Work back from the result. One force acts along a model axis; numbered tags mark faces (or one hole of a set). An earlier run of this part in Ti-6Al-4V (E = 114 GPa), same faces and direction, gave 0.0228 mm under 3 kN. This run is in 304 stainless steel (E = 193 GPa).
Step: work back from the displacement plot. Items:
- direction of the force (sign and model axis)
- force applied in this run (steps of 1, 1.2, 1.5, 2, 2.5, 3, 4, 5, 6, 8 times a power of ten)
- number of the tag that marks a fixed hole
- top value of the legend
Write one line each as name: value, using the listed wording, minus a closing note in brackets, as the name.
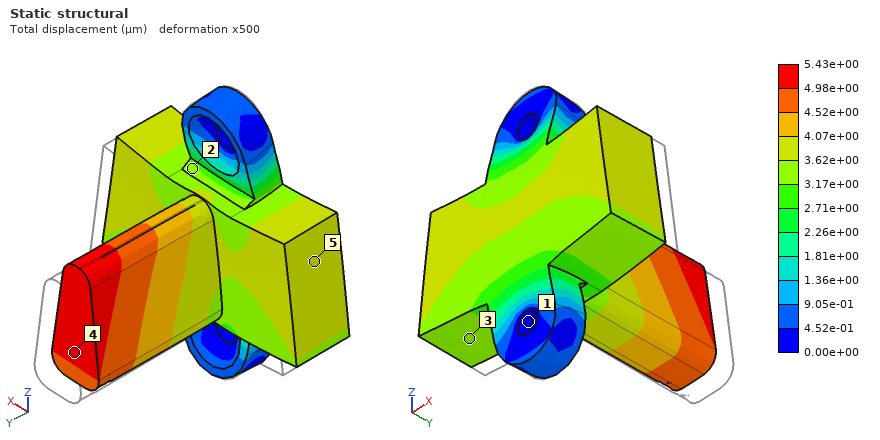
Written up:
direction of the force: -Y
force applied in this run: 1.2 kN
number of the tag that marks a fixed hole: 1
top value of the legend: 5.43e+00 µm
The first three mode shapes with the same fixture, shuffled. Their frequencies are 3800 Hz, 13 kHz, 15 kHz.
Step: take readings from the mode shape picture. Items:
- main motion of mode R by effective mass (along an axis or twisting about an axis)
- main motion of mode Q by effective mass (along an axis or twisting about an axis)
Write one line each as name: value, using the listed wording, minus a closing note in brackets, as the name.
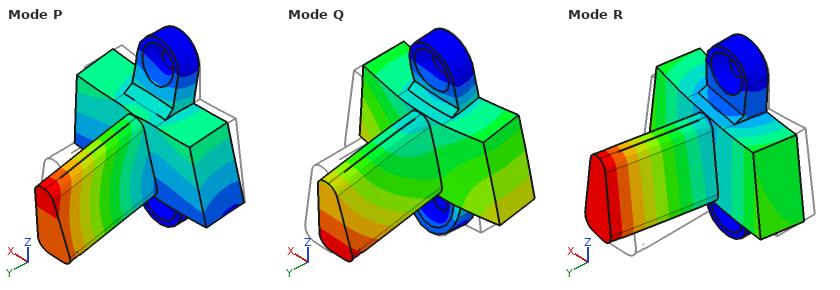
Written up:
main motion of mode R by effective mass: along X
main motion of mode Q by effective mass: along Y
